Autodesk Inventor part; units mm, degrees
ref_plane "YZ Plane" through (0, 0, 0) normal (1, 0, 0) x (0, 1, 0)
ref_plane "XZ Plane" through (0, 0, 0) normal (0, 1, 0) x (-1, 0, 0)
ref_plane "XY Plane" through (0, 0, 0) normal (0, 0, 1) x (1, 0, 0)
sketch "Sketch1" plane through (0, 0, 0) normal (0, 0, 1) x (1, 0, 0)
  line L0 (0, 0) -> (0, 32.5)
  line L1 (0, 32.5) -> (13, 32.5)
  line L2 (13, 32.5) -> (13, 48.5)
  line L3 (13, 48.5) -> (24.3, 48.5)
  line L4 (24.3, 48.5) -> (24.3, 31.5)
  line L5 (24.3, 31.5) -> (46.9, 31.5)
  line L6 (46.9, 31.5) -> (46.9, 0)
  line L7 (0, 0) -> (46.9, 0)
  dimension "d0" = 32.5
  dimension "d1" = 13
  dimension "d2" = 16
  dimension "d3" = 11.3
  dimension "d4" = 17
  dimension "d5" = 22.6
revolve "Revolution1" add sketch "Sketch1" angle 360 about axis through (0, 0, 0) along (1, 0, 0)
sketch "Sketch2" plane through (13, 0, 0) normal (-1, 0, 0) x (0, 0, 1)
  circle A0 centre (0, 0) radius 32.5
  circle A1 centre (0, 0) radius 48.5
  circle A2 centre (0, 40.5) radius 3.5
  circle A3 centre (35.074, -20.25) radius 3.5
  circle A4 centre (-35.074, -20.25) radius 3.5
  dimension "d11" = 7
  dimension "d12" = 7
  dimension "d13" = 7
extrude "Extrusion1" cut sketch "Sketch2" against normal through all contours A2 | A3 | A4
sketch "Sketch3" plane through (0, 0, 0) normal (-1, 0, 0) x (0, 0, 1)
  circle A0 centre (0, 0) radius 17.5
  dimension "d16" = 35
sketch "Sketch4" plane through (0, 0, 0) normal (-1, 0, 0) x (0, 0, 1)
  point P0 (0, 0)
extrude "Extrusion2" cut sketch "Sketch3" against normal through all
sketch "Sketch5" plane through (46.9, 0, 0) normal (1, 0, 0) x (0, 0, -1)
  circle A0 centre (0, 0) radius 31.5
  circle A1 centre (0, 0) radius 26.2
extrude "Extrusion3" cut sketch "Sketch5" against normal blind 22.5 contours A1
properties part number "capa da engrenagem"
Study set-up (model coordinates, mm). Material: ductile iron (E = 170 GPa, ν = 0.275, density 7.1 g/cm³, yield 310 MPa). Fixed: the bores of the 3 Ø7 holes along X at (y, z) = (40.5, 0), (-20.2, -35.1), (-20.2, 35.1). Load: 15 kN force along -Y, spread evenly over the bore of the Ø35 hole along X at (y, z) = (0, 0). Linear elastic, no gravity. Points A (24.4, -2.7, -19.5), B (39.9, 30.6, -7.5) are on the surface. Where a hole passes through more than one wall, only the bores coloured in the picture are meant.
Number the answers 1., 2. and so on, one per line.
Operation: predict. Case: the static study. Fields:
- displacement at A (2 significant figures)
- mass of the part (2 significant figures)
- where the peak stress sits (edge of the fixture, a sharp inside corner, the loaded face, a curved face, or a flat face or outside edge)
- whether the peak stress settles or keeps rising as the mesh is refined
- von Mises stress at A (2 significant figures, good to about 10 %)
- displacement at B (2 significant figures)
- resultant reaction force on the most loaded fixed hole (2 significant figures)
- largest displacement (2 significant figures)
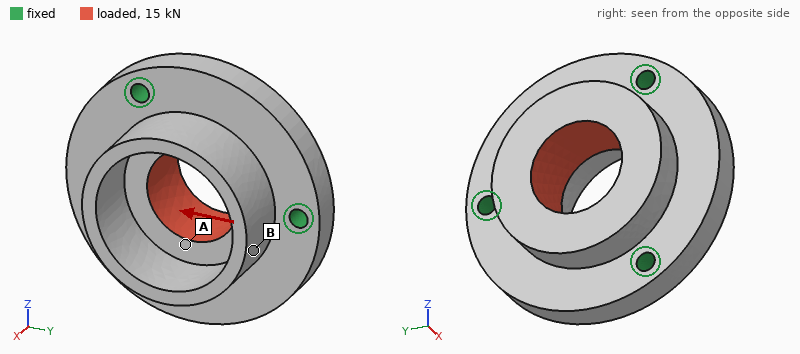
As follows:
1. 2.6 µm
2. 880 g
3. edge of the fixture
4. keeps rising
5. 12 MPa
6. 1.4 µm
7. 5.2 kN
8. 6.6 µm
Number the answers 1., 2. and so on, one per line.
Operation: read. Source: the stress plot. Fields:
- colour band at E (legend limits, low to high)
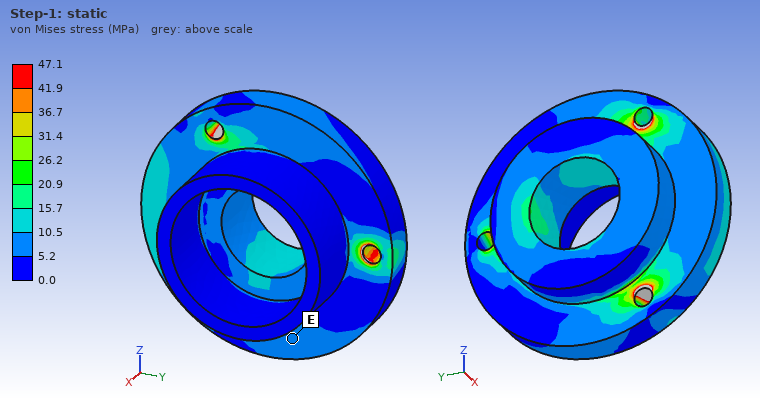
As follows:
1. 5.2 to 10.5 MPa
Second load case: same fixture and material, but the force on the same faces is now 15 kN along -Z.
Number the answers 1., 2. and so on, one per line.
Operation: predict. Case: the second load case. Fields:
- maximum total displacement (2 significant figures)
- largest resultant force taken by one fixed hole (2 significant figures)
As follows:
1. 5.9 µm
2. 5.2 kN
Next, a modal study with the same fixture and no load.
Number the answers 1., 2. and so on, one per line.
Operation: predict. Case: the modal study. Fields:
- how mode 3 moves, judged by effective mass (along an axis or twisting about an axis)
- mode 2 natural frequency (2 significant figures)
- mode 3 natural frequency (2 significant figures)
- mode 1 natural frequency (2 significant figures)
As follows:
1. along X
2. 7200 Hz
3. 8900 Hz
4. 7200 Hz
